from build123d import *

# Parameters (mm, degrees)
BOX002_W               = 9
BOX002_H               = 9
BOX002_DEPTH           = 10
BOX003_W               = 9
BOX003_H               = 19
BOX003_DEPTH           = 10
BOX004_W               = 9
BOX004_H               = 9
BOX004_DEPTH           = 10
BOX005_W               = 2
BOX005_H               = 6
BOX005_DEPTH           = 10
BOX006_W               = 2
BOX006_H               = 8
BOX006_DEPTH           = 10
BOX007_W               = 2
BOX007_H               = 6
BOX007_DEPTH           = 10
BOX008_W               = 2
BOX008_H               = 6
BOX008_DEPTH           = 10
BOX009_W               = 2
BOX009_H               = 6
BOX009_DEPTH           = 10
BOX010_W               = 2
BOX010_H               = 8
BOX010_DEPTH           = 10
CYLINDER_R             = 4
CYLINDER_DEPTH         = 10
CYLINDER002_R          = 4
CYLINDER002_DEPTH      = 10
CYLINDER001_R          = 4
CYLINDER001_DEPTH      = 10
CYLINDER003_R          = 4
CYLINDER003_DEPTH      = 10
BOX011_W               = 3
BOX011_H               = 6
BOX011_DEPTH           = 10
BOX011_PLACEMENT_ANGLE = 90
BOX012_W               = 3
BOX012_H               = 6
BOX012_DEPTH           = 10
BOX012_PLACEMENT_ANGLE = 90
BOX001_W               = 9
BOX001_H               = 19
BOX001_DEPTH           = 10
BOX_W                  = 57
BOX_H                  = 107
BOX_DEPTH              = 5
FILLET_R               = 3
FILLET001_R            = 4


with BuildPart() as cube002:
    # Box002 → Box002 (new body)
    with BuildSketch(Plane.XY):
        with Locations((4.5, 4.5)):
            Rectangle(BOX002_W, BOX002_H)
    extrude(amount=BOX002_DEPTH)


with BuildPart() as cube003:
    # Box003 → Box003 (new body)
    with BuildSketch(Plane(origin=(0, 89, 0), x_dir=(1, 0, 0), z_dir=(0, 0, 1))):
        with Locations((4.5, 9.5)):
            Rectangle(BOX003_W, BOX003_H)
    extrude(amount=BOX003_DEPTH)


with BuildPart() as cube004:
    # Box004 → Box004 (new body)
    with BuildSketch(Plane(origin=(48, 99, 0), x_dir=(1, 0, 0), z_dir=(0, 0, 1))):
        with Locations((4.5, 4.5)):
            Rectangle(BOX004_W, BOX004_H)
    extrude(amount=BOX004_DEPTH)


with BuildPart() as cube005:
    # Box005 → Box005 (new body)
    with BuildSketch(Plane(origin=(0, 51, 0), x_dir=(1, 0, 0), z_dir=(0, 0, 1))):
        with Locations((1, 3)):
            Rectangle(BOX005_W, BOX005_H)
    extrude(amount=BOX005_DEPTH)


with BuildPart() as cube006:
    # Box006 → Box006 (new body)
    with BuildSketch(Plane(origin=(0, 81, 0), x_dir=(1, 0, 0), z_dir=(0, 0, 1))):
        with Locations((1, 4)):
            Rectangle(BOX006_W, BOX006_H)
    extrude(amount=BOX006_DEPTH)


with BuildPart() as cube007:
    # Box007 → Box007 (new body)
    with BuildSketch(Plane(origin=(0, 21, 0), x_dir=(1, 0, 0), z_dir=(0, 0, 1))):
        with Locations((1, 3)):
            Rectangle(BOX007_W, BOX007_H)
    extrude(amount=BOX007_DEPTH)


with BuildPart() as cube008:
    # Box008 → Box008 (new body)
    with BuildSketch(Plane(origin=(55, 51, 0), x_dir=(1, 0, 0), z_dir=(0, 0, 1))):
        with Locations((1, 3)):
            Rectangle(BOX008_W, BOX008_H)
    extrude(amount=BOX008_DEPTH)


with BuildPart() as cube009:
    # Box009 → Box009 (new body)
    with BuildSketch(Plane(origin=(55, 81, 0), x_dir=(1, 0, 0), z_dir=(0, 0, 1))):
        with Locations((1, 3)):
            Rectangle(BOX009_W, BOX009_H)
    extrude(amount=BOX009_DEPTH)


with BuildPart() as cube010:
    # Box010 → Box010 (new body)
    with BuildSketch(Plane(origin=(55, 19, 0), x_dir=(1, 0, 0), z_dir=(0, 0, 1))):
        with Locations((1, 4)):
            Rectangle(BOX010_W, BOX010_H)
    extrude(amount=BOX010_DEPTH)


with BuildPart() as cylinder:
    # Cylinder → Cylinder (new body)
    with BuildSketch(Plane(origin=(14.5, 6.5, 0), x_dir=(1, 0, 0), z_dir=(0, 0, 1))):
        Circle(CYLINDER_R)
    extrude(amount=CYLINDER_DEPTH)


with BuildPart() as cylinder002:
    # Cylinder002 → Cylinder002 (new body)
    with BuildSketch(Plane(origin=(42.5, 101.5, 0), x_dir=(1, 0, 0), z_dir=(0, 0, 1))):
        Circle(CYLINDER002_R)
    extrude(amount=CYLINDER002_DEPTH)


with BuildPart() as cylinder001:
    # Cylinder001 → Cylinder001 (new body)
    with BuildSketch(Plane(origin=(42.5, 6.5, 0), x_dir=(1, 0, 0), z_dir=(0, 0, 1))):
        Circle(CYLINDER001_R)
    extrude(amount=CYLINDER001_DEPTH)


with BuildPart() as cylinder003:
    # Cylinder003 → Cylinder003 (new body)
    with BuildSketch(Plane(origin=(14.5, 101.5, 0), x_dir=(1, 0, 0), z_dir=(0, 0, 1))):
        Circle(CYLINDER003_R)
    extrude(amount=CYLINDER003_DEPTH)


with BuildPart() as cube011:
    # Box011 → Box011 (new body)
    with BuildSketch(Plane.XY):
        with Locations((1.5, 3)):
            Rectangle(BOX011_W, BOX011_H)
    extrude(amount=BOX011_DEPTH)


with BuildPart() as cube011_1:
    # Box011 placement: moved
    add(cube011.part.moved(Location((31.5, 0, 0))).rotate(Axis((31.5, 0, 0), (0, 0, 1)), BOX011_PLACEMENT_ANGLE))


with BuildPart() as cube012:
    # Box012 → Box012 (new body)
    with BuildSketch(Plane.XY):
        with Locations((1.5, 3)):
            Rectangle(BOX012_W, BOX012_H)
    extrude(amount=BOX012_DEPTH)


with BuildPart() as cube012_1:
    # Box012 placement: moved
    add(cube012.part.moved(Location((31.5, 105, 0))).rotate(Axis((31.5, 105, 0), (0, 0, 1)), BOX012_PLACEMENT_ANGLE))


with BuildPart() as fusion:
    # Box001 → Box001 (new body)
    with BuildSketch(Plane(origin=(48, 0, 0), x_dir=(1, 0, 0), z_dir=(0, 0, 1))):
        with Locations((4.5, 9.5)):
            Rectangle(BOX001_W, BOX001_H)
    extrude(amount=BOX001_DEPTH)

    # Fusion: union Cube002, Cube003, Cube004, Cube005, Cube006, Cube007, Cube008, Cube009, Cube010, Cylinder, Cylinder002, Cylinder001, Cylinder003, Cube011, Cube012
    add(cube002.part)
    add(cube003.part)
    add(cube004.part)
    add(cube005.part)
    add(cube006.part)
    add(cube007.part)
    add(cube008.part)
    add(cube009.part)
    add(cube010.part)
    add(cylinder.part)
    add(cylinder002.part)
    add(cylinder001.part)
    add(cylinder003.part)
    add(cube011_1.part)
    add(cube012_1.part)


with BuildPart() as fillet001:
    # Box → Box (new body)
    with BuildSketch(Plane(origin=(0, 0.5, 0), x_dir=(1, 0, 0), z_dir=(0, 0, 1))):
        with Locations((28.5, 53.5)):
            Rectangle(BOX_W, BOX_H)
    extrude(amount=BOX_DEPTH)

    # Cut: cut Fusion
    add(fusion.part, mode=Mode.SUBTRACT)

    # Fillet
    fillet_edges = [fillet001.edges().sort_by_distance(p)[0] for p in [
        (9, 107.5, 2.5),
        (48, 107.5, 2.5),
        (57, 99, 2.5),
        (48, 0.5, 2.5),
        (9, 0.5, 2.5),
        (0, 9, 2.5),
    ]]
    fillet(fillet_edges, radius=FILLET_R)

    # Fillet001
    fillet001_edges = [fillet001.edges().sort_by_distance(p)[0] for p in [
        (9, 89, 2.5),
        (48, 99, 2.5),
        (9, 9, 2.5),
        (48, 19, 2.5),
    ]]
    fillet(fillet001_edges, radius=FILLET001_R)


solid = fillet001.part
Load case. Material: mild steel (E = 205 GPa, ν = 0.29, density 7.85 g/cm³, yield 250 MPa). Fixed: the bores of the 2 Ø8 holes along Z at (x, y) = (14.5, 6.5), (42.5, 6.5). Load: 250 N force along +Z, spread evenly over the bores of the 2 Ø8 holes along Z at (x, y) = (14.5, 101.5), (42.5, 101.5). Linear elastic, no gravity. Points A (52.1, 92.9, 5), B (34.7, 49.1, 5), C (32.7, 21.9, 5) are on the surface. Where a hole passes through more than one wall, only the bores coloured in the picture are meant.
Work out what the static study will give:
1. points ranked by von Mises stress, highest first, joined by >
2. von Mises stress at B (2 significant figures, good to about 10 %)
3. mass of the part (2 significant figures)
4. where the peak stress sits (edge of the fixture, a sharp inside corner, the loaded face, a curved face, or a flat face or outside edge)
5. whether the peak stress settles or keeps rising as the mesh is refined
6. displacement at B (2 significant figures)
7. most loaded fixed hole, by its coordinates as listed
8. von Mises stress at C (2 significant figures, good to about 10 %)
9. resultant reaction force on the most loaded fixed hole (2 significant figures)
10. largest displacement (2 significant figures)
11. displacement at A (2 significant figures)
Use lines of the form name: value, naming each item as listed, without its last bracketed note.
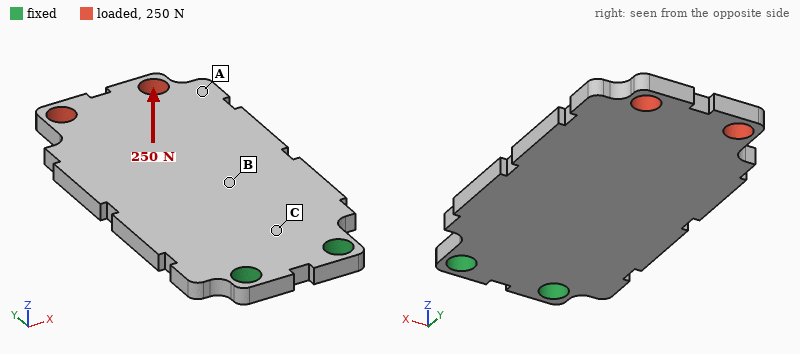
points ranked by von Mises stress, highest first, joined by >: C > B > A
von Mises stress at B: 54 MPa
mass of the part: 210 g
where the peak stress sits: edge of the fixture
whether the peak stress settles or keeps rising as the mesh is refined: keeps rising
displacement at B: 0.16 mm
most loaded fixed hole, by its coordinates as listed: (14.5, 6.5)
von Mises stress at C: 90 MPa
resultant reaction force on the most loaded fixed hole: 160 N
largest displacement: 0.67 mm
displacement at A: 0.53 mm
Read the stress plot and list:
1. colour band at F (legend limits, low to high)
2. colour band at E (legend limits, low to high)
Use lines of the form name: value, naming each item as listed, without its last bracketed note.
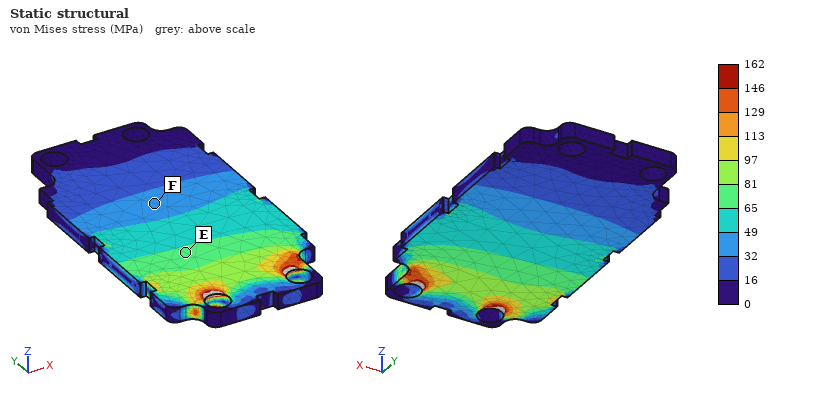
colour band at F: 32 to 49 MPa
colour band at E: 65 to 81 MPa
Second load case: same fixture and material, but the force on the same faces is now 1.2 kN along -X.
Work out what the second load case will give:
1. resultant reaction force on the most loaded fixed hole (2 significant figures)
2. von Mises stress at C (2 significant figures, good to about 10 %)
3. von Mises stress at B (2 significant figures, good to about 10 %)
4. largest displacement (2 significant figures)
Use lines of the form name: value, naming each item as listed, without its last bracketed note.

resultant reaction force on the most loaded fixed hole: 3.7 kN
von Mises stress at C: 26 MPa
von Mises stress at B: 12 MPa
largest displacement: 48 µm
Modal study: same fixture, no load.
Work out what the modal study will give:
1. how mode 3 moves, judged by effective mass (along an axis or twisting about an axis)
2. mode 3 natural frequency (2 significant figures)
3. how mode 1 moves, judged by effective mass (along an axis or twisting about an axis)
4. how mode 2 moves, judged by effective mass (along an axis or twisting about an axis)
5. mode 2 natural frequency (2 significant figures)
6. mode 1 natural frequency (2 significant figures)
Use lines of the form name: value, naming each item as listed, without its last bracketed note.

how mode 3 moves, judged by effective mass: along Z
mode 3 natural frequency: 2700 Hz
how mode 1 moves, judged by effective mass: along Z
how mode 2 moves, judged by effective mass: twisting about Y
mode 2 natural frequency: 1700 Hz
mode 1 natural frequency: 450 Hz
